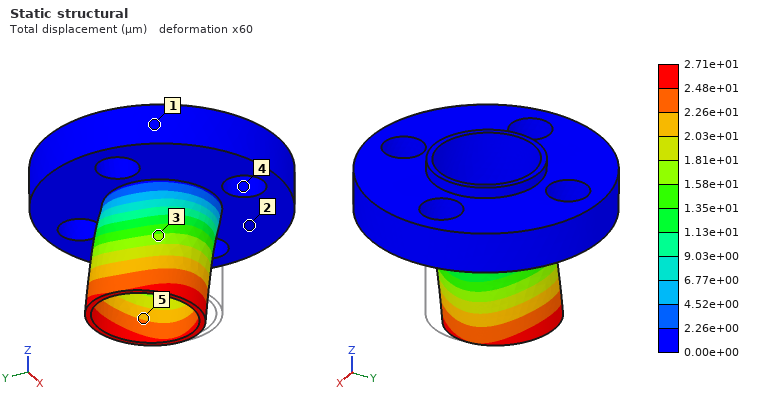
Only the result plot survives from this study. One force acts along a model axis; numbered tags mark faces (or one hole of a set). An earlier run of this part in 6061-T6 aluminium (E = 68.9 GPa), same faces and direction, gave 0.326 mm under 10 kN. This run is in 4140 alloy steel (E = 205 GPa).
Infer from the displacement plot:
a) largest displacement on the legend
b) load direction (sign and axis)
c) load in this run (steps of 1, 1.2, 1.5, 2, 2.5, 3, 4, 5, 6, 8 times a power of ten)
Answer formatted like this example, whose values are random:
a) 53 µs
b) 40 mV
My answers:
a) 2.71e+01 µm
b) +Y
c) 2.5 kN
